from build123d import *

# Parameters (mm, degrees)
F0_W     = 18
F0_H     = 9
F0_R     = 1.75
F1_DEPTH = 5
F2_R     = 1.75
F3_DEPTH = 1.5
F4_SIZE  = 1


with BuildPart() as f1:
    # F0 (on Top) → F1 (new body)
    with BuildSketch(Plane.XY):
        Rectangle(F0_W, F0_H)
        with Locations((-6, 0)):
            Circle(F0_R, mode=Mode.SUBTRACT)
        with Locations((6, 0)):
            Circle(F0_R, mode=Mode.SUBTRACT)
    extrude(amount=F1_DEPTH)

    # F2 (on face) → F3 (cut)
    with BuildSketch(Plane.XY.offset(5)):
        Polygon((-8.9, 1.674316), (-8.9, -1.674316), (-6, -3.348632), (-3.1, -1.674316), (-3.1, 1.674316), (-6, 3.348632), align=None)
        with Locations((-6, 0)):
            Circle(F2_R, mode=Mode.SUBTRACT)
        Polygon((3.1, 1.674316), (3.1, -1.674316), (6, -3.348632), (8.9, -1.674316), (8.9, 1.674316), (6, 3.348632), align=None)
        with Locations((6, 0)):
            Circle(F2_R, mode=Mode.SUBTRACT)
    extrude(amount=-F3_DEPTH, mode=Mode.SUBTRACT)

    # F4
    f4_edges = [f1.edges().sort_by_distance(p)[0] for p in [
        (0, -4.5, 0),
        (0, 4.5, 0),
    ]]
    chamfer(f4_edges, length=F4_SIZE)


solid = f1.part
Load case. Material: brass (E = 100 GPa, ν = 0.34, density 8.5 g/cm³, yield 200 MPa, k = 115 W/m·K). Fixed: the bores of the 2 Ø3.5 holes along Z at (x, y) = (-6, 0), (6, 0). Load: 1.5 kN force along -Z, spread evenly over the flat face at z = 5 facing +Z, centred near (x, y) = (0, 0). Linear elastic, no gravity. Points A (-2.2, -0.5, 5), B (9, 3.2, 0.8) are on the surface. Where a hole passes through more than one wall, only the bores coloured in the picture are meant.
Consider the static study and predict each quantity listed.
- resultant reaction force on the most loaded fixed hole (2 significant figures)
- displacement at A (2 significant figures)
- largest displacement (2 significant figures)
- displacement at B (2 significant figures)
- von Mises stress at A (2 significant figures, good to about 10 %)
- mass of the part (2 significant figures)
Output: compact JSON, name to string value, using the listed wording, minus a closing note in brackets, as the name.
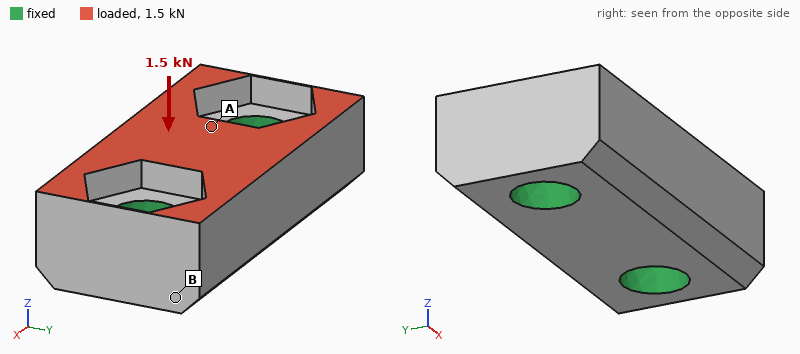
{"resultant reaction force on the most loaded fixed hole": "770 N", "displacement at A": "1.9 µm", "largest displacement": "2.9 µm", "displacement at B": "0.69 µm", "von Mises stress at A": "27 MPa", "mass of the part": "5.4 g"}
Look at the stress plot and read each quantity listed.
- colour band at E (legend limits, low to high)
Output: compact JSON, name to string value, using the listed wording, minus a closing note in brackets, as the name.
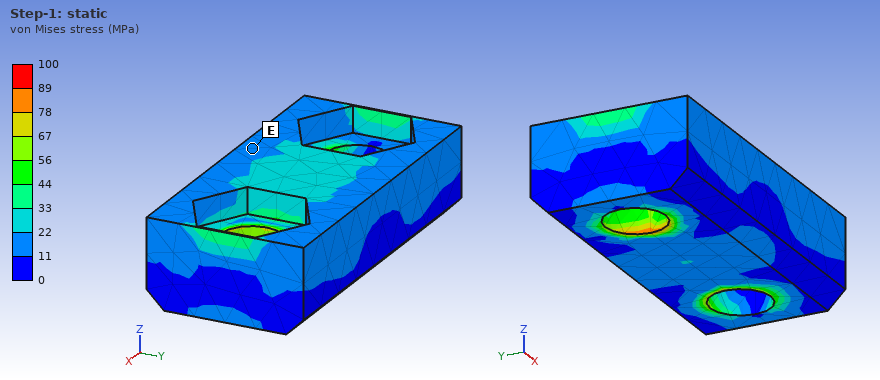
{"colour band at E": "11 to 22 MPa"}
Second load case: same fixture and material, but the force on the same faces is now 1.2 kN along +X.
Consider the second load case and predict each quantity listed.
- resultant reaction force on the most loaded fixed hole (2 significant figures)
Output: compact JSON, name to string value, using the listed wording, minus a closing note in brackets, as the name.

{"resultant reaction force on the most loaded fixed hole": "660 N"}
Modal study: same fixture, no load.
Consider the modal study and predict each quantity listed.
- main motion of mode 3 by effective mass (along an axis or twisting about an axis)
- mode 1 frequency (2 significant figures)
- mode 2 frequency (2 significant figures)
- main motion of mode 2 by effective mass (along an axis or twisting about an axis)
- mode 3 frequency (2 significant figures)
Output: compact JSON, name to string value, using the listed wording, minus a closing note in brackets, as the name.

{"main motion of mode 3 by effective mass": "along Y", "mode 1 frequency": "56 kHz", "mode 2 frequency": "66 kHz", "main motion of mode 2 by effective mass": "along Z", "mode 3 frequency": "80 kHz"}
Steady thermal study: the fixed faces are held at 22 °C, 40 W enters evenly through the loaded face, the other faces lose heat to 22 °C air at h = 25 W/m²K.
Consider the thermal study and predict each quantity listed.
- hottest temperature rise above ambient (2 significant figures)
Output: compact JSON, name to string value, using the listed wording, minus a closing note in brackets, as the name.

{"hottest temperature rise above ambient": "19 K"}
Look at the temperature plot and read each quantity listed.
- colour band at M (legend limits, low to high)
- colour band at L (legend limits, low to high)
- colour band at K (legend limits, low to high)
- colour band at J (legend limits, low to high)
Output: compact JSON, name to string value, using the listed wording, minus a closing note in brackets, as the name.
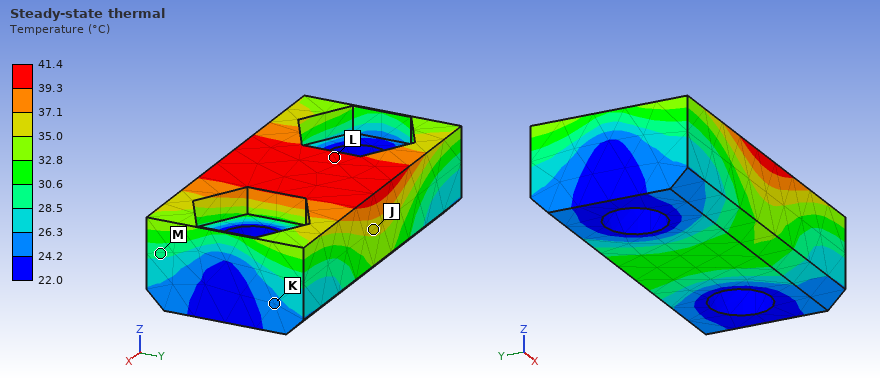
{"colour band at M": "28.5 to 30.6 °C", "colour band at L": "39.3 to 41.4 °C", "colour band at K": "24.2 to 26.3 °C", "colour band at J": "35.0 to 37.1 °C"}
